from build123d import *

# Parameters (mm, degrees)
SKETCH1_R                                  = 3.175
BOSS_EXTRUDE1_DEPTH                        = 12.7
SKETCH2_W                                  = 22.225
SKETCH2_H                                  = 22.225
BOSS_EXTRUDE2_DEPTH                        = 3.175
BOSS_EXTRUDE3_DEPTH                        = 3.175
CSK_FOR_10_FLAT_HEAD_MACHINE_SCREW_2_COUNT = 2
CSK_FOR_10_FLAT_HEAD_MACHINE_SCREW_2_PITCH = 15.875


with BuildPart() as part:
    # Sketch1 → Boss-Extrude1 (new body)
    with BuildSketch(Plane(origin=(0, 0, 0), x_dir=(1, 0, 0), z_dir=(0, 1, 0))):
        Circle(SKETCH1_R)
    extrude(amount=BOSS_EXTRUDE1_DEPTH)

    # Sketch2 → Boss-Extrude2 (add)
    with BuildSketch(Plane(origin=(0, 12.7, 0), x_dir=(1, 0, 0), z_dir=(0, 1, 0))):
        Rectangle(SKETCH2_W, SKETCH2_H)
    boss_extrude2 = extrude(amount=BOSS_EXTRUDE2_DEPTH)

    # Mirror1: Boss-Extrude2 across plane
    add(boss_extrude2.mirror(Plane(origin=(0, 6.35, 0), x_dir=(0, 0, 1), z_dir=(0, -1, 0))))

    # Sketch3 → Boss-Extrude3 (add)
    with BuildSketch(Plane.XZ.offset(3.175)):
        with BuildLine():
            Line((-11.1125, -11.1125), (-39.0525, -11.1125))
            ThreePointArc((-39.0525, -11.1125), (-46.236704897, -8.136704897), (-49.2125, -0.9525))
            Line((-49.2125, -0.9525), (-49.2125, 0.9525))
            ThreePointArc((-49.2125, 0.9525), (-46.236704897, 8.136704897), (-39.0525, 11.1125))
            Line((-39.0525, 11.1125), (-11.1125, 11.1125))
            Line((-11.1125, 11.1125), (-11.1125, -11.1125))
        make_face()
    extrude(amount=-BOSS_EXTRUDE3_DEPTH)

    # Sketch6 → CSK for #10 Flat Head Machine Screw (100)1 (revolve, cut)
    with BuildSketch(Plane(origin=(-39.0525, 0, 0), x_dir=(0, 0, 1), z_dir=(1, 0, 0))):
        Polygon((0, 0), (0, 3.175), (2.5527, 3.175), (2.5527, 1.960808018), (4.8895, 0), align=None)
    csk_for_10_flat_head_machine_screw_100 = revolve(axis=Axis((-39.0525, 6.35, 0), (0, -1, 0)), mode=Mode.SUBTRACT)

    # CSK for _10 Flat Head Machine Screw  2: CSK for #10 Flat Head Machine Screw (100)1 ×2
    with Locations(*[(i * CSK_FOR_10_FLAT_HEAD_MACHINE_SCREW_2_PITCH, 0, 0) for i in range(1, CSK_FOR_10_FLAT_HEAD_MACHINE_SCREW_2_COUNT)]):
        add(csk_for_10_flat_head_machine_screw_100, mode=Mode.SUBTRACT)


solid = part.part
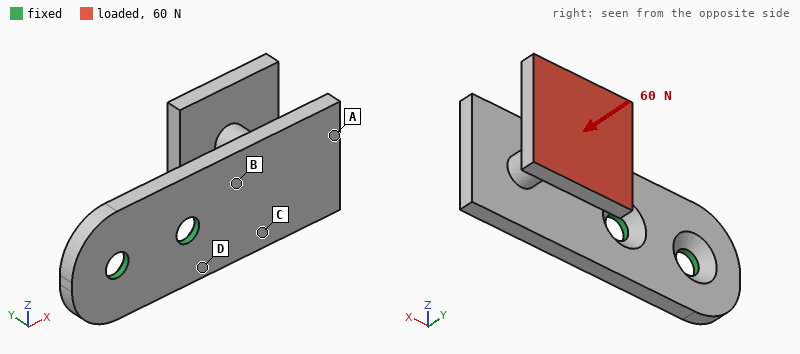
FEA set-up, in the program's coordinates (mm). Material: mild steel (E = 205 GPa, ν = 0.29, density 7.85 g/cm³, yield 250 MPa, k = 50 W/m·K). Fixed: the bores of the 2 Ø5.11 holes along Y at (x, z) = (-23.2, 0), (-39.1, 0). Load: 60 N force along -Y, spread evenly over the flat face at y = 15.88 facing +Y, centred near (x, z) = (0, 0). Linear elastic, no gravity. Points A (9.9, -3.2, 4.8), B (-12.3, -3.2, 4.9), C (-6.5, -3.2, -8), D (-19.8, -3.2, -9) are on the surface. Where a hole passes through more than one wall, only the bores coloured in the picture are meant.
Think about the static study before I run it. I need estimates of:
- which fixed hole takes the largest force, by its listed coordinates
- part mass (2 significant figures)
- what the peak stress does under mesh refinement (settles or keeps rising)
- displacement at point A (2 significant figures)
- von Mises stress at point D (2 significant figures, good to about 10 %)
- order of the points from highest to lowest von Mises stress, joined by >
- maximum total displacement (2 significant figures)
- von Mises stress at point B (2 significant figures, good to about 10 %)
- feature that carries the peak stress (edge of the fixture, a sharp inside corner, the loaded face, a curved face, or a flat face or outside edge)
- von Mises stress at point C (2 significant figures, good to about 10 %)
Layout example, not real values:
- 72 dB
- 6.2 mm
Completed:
- (-23.2, 0)
- 46 g
- keeps rising
- 43 µm
- 27 MPa
- D > B > C > A
- 54 µm
- 19 MPa
- edge of the fixture
- 10 MPa
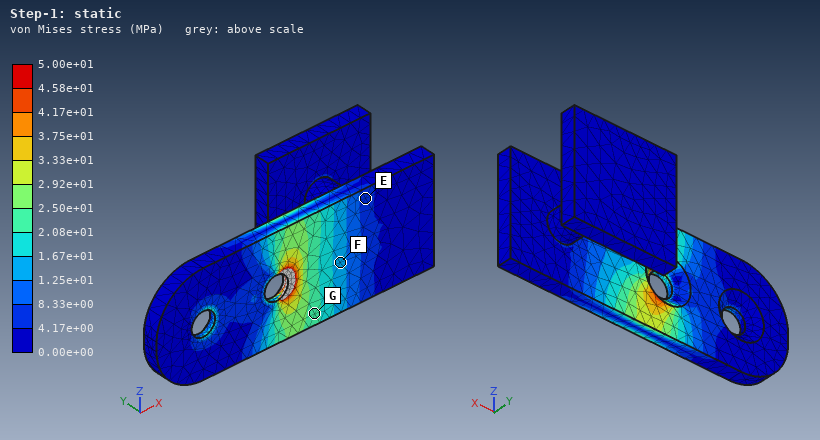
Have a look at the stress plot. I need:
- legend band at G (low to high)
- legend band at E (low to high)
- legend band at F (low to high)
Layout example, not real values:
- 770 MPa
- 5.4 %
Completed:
- 2.08e+01 to 2.50e+01 MPa
- 4.17e+00 to 8.33e+00 MPa
- 1.25e+01 to 1.67e+01 MPa
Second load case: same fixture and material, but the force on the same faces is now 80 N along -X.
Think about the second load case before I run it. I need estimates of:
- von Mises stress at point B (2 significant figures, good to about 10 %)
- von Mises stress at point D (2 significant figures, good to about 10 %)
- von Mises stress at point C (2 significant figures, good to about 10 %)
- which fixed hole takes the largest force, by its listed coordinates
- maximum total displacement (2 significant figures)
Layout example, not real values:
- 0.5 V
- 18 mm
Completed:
- 34 MPa
- 33 MPa
- 34 MPa
- (-39.1, 0)
- 98 µm
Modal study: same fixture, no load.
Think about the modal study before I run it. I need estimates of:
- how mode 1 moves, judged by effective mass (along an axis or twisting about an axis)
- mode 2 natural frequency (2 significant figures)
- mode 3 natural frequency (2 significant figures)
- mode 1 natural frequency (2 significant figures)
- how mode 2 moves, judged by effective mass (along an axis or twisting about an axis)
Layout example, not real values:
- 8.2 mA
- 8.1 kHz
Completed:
- along Y
- 1700 Hz
- 3500 Hz
- 1100 Hz
- along Z
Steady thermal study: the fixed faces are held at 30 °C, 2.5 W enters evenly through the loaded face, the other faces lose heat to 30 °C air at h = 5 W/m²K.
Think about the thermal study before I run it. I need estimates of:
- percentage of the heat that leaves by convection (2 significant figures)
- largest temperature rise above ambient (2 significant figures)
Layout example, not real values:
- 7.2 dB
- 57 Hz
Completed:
- 12 %
- 41 K
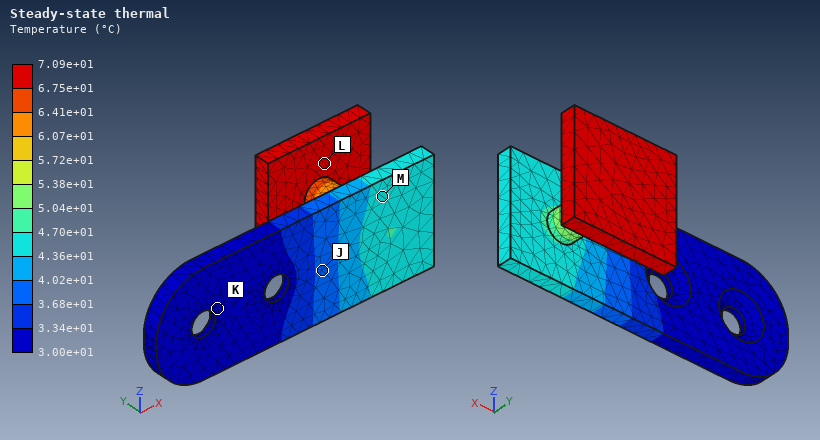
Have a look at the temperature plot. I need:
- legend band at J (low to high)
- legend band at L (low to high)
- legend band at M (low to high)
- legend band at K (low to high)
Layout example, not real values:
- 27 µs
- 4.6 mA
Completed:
- 3.68e+01 to 4.02e+01 °C
- 6.75e+01 to 7.09e+01 °C
- 4.36e+01 to 4.70e+01 °C
- 3.00e+01 to 3.34e+01 °C
